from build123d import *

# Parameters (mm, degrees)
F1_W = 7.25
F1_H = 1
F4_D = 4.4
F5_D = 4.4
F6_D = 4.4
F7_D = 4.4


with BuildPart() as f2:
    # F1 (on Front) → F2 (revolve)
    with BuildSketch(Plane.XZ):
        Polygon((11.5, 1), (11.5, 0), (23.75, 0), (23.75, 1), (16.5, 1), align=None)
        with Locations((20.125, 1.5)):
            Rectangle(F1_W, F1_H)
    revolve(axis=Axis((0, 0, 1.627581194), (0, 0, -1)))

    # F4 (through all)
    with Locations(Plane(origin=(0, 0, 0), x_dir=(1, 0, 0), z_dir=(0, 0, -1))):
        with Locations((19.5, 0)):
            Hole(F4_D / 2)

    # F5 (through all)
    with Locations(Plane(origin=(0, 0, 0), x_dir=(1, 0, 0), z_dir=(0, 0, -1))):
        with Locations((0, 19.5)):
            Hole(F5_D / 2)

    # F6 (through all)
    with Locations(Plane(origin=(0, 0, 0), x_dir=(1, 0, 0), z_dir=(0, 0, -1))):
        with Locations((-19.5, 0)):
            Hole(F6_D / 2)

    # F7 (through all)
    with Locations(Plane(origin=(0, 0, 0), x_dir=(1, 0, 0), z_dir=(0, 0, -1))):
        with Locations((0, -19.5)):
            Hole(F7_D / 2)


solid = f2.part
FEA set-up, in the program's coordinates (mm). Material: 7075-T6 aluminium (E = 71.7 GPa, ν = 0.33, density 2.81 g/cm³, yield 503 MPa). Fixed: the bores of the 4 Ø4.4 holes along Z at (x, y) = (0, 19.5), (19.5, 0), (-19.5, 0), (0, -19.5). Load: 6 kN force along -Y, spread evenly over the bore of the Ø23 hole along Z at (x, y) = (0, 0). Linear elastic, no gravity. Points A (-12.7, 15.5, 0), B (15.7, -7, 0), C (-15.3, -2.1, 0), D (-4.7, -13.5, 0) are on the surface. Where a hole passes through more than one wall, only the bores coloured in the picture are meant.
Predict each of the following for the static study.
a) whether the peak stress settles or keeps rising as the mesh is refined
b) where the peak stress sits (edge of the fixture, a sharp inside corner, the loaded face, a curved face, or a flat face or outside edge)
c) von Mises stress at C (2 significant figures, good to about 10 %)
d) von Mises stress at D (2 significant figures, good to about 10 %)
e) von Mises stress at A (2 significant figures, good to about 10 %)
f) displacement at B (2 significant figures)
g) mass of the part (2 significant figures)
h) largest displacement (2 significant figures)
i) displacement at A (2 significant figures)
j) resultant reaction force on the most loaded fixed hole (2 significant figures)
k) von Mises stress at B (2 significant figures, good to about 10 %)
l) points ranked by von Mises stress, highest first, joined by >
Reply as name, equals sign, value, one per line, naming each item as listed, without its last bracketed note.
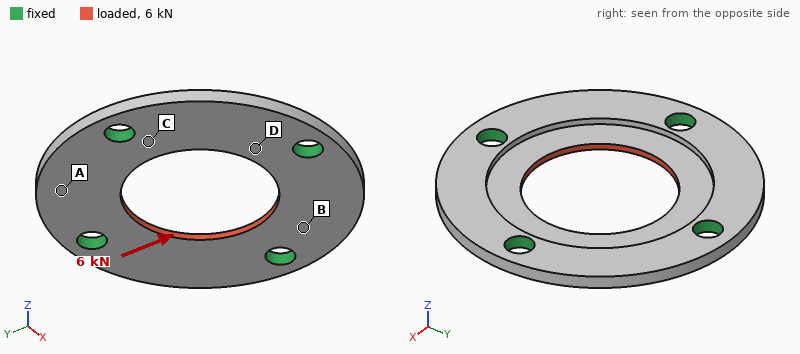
whether the peak stress settles or keeps rising as the mesh is refined = keeps rising
where the peak stress sits = edge of the fixture
von Mises stress at C = 85 MPa
von Mises stress at D = 120 MPa
von Mises stress at A = 39 MPa
displacement at B = 11 µm
mass of the part = 6.0 g
largest displacement = 29 µm
displacement at A = 17 µm
resultant reaction force on the most loaded fixed hole = 1.6 kN
von Mises stress at B = 61 MPa
points ranked by von Mises stress, highest first, joined by > = D > C > B > A
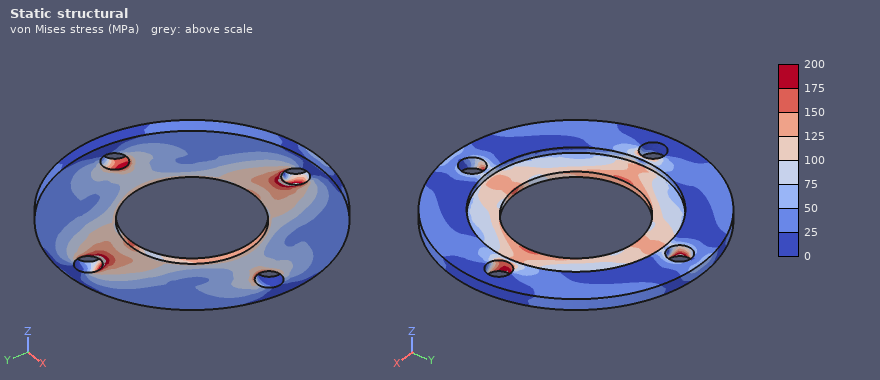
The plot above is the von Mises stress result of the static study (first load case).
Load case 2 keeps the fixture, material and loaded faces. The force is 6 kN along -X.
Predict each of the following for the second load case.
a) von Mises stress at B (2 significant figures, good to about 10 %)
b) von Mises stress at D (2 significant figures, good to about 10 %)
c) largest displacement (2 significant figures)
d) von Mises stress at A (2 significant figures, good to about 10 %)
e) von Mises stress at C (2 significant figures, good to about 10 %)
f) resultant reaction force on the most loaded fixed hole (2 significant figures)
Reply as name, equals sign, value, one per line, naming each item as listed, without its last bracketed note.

von Mises stress at B = 83 MPa
von Mises stress at D = 66 MPa
largest displacement = 29 µm
von Mises stress at A = 40 MPa
von Mises stress at C = 140 MPa
resultant reaction force on the most loaded fixed hole = 1.6 kN
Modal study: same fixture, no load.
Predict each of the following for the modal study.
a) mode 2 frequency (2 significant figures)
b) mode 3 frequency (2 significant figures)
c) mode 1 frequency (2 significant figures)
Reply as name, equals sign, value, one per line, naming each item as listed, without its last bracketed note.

mode 2 frequency = 12 kHz
mode 3 frequency = 12 kHz
mode 1 frequency = 12 kHz
